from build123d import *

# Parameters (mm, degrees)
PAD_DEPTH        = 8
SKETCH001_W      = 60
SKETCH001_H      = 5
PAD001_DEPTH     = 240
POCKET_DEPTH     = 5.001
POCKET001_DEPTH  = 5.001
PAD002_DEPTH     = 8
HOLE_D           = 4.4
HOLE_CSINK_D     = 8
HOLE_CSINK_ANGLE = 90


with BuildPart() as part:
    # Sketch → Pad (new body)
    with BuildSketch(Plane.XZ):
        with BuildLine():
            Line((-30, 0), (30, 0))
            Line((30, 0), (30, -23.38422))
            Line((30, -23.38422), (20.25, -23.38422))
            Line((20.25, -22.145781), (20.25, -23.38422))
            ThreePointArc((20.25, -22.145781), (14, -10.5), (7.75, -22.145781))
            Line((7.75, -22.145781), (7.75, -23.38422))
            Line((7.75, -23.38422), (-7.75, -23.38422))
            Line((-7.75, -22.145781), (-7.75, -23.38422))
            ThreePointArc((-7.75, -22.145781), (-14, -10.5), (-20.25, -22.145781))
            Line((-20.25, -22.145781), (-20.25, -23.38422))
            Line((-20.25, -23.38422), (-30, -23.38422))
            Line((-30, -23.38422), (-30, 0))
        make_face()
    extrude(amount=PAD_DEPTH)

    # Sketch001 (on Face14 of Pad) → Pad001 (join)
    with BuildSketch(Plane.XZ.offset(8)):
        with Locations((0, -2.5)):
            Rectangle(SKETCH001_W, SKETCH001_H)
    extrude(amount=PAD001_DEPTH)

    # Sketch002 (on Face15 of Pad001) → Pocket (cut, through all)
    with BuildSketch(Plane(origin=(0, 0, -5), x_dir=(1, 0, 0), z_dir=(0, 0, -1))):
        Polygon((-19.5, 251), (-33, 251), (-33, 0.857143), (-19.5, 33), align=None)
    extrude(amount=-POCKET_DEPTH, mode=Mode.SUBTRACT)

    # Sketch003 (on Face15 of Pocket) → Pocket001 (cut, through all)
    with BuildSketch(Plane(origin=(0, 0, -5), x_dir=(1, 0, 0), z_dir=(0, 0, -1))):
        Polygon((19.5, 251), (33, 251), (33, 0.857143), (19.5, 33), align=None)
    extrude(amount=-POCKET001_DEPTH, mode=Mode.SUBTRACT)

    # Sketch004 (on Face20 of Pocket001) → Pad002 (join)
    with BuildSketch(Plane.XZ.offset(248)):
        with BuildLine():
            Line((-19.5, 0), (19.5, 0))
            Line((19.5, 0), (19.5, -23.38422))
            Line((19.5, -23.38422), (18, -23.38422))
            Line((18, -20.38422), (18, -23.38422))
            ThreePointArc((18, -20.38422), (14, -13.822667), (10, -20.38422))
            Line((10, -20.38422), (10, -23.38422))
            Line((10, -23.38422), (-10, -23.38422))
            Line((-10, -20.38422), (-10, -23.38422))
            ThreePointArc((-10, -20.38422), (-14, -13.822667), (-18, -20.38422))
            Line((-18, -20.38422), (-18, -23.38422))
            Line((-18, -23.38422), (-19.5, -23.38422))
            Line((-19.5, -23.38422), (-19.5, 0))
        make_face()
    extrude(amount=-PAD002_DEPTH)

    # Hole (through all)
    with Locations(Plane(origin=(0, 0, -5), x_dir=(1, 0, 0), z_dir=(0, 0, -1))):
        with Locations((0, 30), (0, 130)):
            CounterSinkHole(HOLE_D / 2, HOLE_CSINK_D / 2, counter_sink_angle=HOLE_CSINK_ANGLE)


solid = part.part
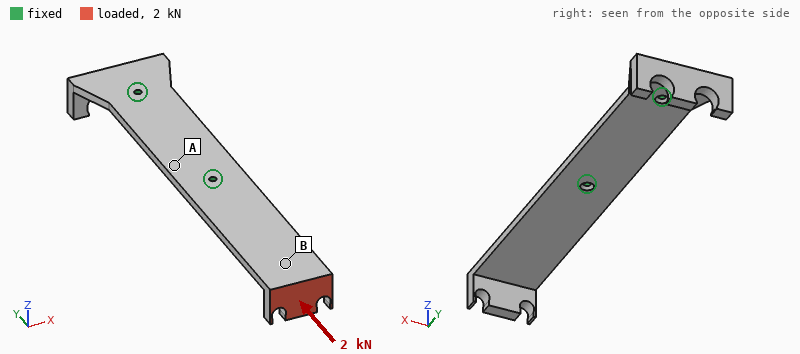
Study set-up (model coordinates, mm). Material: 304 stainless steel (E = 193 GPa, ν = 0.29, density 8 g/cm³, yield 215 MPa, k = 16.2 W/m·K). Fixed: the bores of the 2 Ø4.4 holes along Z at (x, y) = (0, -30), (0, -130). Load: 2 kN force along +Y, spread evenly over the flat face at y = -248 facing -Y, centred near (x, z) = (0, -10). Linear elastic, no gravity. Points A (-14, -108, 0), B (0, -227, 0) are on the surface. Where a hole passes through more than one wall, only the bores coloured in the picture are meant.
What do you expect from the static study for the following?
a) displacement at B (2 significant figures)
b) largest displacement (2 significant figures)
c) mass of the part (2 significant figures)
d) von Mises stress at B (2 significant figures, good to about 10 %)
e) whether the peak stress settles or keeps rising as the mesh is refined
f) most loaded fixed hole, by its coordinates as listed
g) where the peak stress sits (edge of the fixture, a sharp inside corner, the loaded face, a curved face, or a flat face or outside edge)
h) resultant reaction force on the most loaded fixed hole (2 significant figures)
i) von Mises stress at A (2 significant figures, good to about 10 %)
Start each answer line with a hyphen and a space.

- 1.0 mm
- 1.6 mm
- 490 g
- 77 MPa
- keeps rising
- (0, -130)
- edge of the fixture
- 1.4 kN
- 15 MPa
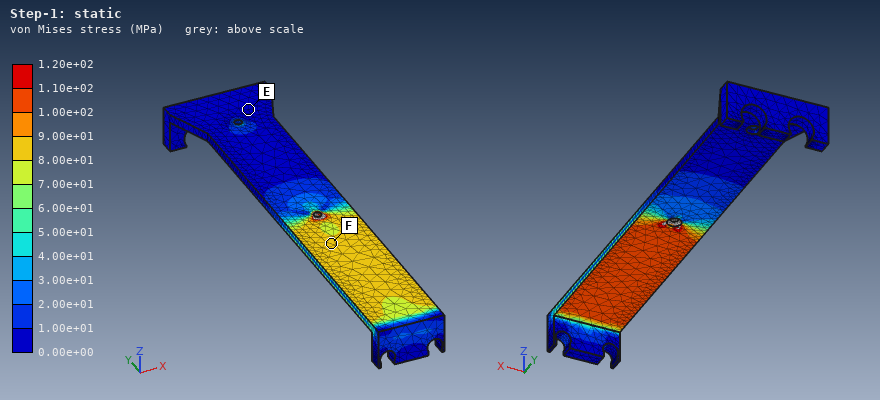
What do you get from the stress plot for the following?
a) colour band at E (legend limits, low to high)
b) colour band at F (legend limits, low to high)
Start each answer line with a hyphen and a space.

- 0.00e+00 to 1.00e+01 MPa
- 8.00e+01 to 9.00e+01 MPa
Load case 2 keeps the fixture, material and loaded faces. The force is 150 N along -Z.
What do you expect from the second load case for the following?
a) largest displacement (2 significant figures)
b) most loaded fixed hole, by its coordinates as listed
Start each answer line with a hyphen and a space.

- 1.2 mm
- (0, -130)
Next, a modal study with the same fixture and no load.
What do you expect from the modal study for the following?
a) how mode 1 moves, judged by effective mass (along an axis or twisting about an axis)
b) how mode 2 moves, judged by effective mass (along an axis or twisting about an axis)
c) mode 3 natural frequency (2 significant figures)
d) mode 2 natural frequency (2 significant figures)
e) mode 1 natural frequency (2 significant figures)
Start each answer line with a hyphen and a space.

- along Z
- along X
- 1300 Hz
- 1000 Hz
- 200 Hz
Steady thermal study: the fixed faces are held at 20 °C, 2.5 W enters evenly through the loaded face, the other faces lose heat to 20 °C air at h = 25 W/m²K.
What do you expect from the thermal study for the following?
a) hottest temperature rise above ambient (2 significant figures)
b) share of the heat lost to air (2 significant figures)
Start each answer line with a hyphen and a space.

- 23 K
- 95 %
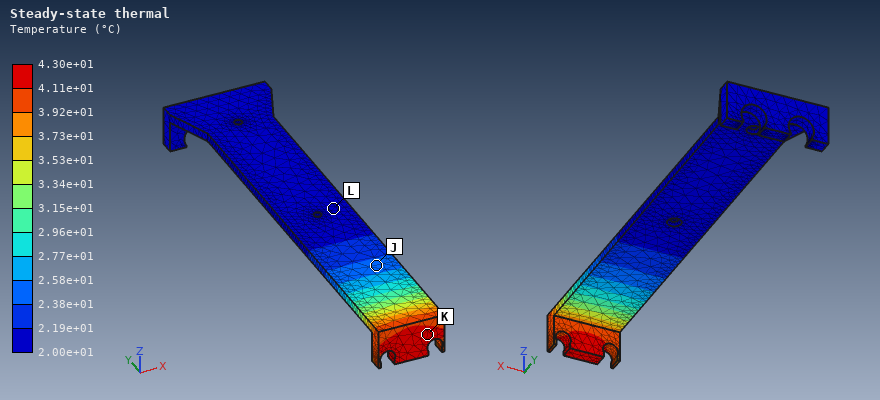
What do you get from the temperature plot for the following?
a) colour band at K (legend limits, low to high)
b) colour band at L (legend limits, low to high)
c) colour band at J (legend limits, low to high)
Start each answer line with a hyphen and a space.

- 4.11e+01 to 4.30e+01 °C
- 2.00e+01 to 2.19e+01 °C
- 2.38e+01 to 2.58e+01 °C
